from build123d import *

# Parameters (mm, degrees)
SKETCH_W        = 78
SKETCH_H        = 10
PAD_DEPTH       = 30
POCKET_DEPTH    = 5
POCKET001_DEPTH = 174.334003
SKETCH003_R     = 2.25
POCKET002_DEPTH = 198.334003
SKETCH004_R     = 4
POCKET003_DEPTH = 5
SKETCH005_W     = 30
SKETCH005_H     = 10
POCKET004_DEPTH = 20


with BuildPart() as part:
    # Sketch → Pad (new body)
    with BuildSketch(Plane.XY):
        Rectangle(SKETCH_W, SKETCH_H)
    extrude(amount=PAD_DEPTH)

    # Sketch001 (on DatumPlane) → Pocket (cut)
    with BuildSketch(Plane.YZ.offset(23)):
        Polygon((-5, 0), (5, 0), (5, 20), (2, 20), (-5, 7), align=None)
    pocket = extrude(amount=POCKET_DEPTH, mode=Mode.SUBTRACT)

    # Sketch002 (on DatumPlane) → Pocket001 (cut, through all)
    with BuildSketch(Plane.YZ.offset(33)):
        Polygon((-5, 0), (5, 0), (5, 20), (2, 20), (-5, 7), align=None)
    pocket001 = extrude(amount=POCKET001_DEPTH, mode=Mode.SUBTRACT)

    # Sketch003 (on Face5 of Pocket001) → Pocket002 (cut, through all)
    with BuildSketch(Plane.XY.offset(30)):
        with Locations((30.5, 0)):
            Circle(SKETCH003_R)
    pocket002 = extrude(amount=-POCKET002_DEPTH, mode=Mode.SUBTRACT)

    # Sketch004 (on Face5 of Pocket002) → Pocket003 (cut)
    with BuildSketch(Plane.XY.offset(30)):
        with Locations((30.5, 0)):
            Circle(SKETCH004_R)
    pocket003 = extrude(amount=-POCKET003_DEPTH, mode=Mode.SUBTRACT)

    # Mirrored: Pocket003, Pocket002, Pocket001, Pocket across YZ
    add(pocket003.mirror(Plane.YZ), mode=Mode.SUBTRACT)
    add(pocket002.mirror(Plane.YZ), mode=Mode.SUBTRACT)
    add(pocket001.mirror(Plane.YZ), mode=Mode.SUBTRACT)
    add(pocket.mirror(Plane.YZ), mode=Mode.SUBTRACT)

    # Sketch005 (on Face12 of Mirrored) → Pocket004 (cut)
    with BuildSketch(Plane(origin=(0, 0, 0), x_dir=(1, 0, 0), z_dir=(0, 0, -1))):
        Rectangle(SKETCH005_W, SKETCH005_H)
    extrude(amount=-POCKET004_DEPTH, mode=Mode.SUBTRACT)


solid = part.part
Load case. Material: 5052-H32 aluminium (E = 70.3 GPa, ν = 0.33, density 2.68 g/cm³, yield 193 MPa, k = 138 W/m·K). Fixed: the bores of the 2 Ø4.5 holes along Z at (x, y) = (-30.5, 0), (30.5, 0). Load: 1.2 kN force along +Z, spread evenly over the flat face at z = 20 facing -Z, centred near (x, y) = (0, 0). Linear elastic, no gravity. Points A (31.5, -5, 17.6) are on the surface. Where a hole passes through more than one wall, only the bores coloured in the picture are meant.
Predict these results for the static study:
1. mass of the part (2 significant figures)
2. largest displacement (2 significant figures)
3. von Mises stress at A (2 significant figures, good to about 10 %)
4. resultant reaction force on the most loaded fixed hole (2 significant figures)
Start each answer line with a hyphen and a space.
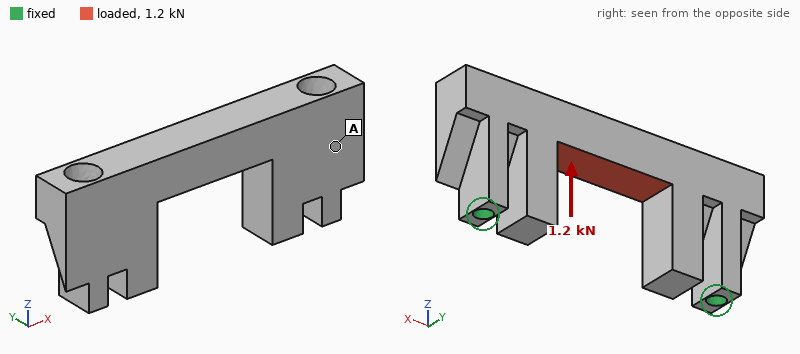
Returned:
- 34 g
- 16 µm
- 5.0 MPa
- 760 N
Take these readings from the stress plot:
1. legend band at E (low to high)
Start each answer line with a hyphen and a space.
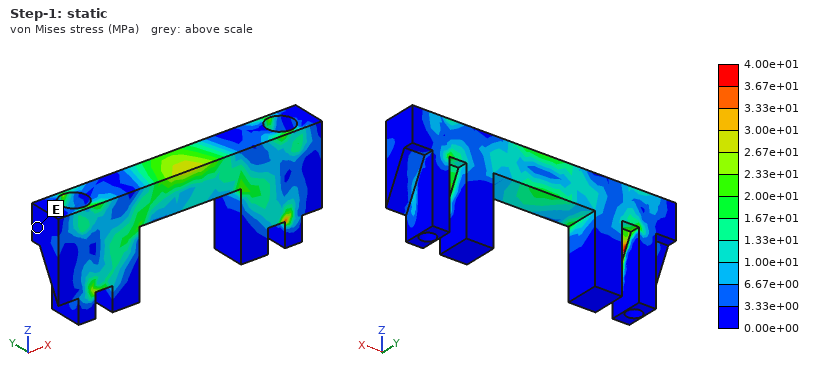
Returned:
- 0.00e+00 to 3.33e+00 MPa
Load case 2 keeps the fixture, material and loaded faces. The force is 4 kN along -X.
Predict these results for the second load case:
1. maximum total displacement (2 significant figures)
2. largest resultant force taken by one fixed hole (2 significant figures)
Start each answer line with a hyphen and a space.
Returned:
- 12 µm
- 2.0 kN
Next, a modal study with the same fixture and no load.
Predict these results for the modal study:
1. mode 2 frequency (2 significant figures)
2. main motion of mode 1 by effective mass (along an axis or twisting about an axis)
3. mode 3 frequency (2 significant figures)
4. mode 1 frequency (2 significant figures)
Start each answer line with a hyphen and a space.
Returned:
- 11 kHz
- along Y
- 12 kHz
- 9600 Hz
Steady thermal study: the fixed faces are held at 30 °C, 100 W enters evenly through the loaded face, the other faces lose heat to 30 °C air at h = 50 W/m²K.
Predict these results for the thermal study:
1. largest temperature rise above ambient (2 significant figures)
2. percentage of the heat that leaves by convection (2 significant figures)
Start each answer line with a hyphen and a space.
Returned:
- 75 K
- 5.6 %
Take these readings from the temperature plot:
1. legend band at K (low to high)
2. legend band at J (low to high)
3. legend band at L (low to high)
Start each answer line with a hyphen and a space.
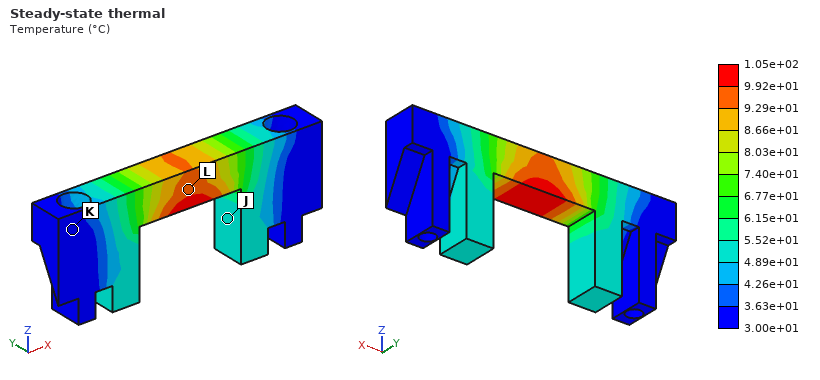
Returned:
- 3.00e+01 to 3.63e+01 °C
- 4.89e+01 to 5.52e+01 °C
- 9.29e+01 to 9.92e+01 °C
